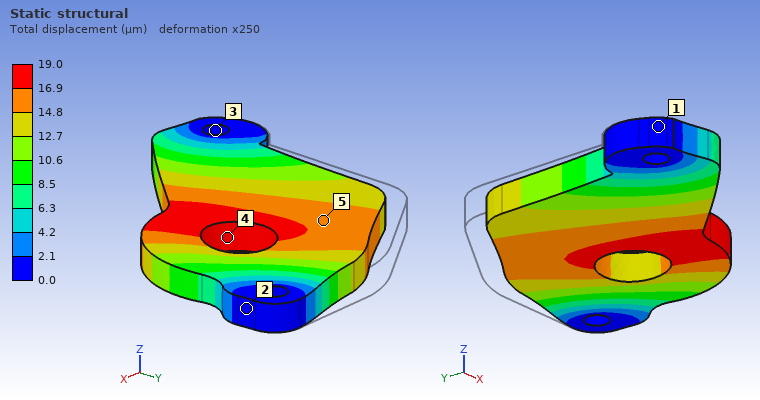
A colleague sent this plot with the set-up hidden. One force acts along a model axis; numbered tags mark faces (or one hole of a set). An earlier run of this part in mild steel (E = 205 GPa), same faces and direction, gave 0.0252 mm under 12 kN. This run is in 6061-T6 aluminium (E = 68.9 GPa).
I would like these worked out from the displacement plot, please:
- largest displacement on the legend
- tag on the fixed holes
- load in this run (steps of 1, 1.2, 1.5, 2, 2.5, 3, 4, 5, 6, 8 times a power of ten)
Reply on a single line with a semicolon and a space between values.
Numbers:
19.0 µm; 3; 3 kN
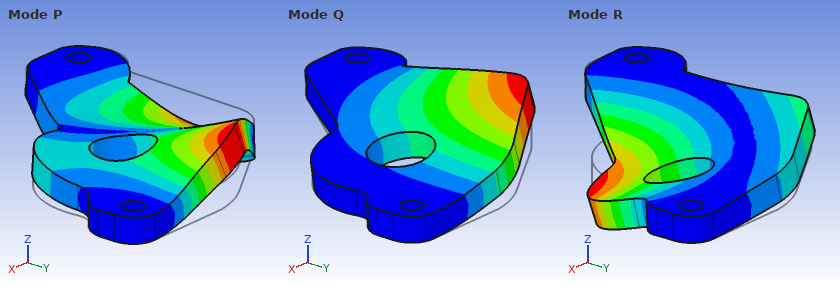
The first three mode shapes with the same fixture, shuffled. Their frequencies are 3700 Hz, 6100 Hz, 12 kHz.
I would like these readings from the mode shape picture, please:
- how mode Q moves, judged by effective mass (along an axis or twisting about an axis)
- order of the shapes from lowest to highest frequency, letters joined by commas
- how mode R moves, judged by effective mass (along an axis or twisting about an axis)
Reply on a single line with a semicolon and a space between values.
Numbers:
along Z; Q, R, P; along Z
